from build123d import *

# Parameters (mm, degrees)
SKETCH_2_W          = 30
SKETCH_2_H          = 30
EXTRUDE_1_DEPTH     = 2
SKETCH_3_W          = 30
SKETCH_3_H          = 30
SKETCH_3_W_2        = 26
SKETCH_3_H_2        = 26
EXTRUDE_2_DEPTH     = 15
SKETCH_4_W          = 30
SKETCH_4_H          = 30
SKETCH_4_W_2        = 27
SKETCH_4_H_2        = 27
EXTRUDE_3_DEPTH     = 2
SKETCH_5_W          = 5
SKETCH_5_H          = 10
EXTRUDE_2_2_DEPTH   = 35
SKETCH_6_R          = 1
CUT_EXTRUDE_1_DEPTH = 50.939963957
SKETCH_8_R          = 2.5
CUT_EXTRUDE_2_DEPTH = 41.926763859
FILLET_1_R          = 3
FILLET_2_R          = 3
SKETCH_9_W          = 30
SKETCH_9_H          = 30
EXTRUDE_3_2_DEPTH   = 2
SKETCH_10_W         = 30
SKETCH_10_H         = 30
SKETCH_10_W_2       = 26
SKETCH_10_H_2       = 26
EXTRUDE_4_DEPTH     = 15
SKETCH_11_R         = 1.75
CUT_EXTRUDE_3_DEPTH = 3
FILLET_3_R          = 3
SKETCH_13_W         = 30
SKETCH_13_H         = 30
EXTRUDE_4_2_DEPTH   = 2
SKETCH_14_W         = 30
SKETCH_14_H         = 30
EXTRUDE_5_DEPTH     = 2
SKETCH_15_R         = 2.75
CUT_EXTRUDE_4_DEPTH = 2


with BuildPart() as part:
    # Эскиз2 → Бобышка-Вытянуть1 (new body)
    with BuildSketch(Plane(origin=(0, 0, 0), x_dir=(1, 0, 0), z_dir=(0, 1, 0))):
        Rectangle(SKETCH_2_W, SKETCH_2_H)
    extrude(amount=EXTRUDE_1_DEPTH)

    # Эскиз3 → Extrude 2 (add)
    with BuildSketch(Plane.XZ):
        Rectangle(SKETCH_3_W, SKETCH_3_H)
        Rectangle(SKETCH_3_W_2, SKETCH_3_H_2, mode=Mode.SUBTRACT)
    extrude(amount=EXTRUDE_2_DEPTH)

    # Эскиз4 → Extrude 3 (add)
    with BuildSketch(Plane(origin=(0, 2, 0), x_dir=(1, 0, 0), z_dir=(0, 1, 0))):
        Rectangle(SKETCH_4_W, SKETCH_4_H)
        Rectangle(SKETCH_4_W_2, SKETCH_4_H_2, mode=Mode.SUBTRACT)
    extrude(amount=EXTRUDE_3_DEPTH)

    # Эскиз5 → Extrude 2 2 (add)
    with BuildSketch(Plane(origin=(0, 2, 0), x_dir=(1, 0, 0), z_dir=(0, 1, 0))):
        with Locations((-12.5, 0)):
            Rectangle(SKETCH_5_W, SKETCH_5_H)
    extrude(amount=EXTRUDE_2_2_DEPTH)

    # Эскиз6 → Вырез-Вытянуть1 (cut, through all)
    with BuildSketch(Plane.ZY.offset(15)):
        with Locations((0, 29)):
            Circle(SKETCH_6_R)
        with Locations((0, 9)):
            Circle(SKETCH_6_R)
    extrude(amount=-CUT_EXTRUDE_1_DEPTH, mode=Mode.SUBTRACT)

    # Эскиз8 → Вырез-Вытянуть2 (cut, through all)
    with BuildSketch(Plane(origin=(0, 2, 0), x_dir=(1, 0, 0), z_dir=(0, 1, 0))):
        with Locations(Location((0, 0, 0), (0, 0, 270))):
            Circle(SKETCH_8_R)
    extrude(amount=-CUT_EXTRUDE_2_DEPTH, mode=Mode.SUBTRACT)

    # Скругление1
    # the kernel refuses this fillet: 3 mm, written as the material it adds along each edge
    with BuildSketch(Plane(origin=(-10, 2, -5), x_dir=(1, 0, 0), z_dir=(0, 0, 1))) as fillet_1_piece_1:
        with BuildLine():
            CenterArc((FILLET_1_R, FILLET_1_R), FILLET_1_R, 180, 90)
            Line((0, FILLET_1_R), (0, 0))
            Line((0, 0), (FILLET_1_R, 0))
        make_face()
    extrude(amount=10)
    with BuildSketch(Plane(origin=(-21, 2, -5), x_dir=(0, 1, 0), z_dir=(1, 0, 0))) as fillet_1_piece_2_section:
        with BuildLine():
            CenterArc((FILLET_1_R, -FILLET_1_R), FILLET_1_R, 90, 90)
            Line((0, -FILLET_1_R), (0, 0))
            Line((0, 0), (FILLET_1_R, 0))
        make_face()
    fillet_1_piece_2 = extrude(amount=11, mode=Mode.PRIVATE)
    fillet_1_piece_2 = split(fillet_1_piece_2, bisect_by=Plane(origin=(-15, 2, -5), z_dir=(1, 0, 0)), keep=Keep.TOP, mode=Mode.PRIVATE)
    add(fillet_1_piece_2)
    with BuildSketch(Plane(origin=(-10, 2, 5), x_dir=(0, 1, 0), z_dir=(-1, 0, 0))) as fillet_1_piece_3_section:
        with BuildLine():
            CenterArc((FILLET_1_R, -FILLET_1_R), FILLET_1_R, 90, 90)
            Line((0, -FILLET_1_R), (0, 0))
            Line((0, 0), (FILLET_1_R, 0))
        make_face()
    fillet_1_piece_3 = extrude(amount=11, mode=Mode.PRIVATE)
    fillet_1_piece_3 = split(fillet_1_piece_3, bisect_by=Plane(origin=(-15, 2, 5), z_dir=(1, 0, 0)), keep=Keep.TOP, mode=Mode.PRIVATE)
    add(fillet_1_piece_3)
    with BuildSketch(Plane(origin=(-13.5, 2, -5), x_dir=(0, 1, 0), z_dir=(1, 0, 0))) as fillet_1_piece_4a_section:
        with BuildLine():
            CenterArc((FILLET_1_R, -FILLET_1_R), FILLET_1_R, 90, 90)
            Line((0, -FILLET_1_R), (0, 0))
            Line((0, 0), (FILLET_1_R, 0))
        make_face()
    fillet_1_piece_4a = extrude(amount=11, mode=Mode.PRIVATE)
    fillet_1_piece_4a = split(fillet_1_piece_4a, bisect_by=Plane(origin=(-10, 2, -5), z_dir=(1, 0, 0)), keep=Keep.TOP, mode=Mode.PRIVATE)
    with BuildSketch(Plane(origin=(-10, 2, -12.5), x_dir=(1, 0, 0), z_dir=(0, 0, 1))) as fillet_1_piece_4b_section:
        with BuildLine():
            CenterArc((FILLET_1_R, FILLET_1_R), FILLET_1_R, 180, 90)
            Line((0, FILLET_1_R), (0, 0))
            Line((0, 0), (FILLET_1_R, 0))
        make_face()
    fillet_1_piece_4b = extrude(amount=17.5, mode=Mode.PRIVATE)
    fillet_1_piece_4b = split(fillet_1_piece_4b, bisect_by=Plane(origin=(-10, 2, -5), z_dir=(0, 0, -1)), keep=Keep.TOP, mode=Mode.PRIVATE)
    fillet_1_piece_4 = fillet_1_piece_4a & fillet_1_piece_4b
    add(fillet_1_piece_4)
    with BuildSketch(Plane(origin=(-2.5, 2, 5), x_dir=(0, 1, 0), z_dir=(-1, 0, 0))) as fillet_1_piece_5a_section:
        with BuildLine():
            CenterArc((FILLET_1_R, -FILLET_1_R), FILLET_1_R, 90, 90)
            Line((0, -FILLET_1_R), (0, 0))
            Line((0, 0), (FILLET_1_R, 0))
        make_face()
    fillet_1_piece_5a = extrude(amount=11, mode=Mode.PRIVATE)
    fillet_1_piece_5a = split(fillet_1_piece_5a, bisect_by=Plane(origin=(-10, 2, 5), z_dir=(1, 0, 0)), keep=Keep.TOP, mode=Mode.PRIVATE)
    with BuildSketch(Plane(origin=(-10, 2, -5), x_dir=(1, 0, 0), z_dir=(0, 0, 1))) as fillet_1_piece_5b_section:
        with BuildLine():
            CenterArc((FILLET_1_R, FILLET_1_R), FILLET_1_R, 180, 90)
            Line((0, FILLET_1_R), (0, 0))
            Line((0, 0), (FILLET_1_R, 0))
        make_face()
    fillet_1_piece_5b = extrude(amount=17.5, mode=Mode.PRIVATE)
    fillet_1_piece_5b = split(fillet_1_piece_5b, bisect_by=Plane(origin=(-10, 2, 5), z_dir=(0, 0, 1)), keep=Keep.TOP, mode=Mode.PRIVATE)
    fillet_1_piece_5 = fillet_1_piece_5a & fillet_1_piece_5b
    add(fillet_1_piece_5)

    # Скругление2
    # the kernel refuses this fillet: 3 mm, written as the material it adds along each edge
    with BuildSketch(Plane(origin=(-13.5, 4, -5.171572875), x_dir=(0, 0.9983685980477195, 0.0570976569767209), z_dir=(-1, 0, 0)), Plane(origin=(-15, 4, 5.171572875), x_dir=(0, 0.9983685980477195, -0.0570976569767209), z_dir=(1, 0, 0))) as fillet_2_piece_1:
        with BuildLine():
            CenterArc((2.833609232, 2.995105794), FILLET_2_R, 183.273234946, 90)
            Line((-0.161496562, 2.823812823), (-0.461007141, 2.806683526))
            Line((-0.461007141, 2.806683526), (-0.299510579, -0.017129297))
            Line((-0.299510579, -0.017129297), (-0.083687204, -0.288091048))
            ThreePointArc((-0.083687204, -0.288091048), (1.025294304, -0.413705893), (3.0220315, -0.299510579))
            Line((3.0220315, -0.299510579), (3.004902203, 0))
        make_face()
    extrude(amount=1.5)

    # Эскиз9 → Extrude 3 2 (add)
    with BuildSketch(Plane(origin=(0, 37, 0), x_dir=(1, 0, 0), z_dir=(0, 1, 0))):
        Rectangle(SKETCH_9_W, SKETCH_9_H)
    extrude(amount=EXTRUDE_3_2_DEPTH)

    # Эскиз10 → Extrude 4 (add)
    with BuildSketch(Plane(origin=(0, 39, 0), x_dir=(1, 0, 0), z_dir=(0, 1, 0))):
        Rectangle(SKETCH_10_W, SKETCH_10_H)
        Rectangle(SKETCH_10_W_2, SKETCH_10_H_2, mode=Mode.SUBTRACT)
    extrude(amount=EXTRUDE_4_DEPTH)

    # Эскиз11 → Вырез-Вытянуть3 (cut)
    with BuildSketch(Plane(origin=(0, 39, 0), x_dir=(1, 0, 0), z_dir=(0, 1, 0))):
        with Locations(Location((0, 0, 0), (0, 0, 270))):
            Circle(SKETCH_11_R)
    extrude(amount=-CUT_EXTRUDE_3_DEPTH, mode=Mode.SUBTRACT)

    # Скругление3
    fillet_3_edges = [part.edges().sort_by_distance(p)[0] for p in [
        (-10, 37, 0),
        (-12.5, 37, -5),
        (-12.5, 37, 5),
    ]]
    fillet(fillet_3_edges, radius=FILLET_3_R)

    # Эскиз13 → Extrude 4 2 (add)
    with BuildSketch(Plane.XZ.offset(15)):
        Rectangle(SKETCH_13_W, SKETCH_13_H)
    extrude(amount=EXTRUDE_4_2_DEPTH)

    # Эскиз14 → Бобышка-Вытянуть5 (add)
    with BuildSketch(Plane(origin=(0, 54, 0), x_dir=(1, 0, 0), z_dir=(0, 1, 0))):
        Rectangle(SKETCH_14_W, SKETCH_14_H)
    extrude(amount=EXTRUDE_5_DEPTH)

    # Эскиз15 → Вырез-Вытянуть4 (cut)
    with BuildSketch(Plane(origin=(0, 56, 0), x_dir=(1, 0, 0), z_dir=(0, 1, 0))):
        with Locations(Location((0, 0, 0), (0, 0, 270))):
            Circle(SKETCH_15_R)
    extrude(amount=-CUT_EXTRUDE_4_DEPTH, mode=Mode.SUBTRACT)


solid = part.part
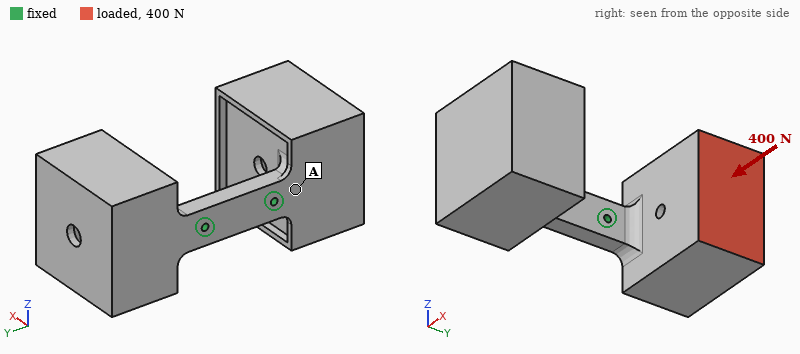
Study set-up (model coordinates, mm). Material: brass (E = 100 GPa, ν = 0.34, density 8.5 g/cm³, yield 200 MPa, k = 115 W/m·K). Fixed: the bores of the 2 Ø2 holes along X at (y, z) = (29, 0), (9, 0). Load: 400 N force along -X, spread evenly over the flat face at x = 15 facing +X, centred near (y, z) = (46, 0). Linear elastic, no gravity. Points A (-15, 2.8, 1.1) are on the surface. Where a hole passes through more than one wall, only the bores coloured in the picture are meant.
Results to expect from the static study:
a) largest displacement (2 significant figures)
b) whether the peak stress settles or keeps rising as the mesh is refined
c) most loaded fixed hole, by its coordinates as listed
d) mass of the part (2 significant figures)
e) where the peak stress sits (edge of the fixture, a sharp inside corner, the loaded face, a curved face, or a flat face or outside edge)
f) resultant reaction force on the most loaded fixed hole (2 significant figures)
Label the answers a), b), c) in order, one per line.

a) 0.25 mm
b) keeps rising
c) (29, 0)
d) 140 g
e) edge of the fixture
f) 480 N
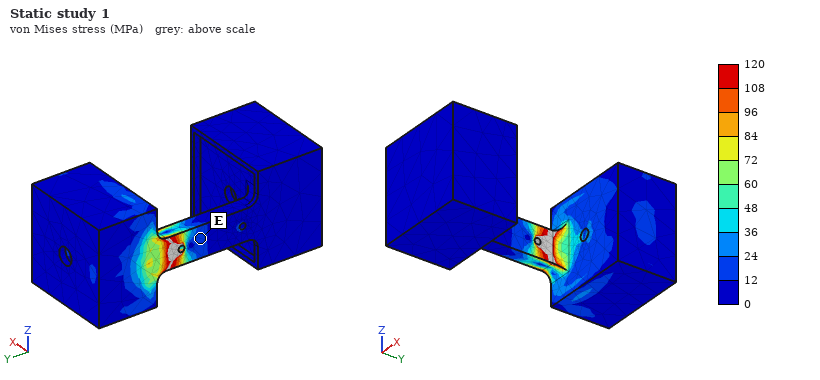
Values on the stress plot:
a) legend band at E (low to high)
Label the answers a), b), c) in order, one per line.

a) 12 to 24 MPa
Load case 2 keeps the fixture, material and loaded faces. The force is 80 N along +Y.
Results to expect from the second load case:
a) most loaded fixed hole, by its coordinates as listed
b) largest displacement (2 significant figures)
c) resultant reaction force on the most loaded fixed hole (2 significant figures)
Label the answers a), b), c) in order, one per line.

a) (29, 0)
b) 0.12 mm
c) 77 N
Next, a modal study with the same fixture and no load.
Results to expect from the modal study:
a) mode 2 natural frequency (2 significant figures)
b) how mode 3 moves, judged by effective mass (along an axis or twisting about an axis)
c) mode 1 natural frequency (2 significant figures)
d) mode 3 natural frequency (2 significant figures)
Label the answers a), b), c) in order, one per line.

a) 820 Hz
b) along Z
c) 790 Hz
d) 1100 Hz
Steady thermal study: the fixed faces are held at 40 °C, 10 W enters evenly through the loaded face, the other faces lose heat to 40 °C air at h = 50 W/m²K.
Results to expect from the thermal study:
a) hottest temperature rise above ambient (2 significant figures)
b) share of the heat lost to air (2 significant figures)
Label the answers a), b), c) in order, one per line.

a) 23 K
b) 49 %
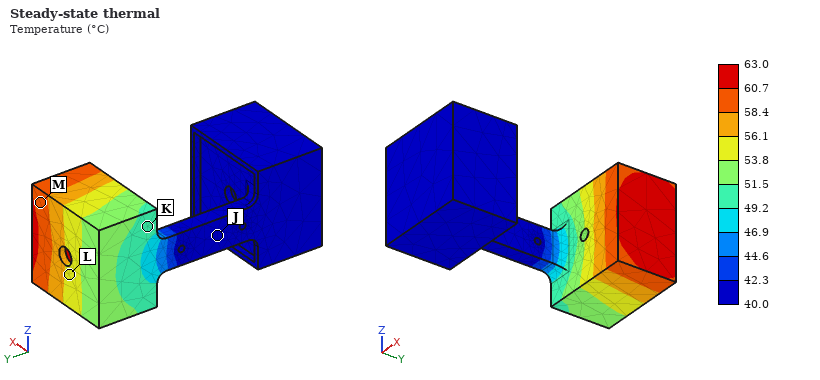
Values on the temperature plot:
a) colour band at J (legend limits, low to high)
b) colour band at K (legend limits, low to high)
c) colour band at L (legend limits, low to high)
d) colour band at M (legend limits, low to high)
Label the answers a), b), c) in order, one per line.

a) 40.0 to 42.3 °C
b) 49.2 to 51.5 °C
c) 53.8 to 56.1 °C
d) 58.4 to 60.7 °C
